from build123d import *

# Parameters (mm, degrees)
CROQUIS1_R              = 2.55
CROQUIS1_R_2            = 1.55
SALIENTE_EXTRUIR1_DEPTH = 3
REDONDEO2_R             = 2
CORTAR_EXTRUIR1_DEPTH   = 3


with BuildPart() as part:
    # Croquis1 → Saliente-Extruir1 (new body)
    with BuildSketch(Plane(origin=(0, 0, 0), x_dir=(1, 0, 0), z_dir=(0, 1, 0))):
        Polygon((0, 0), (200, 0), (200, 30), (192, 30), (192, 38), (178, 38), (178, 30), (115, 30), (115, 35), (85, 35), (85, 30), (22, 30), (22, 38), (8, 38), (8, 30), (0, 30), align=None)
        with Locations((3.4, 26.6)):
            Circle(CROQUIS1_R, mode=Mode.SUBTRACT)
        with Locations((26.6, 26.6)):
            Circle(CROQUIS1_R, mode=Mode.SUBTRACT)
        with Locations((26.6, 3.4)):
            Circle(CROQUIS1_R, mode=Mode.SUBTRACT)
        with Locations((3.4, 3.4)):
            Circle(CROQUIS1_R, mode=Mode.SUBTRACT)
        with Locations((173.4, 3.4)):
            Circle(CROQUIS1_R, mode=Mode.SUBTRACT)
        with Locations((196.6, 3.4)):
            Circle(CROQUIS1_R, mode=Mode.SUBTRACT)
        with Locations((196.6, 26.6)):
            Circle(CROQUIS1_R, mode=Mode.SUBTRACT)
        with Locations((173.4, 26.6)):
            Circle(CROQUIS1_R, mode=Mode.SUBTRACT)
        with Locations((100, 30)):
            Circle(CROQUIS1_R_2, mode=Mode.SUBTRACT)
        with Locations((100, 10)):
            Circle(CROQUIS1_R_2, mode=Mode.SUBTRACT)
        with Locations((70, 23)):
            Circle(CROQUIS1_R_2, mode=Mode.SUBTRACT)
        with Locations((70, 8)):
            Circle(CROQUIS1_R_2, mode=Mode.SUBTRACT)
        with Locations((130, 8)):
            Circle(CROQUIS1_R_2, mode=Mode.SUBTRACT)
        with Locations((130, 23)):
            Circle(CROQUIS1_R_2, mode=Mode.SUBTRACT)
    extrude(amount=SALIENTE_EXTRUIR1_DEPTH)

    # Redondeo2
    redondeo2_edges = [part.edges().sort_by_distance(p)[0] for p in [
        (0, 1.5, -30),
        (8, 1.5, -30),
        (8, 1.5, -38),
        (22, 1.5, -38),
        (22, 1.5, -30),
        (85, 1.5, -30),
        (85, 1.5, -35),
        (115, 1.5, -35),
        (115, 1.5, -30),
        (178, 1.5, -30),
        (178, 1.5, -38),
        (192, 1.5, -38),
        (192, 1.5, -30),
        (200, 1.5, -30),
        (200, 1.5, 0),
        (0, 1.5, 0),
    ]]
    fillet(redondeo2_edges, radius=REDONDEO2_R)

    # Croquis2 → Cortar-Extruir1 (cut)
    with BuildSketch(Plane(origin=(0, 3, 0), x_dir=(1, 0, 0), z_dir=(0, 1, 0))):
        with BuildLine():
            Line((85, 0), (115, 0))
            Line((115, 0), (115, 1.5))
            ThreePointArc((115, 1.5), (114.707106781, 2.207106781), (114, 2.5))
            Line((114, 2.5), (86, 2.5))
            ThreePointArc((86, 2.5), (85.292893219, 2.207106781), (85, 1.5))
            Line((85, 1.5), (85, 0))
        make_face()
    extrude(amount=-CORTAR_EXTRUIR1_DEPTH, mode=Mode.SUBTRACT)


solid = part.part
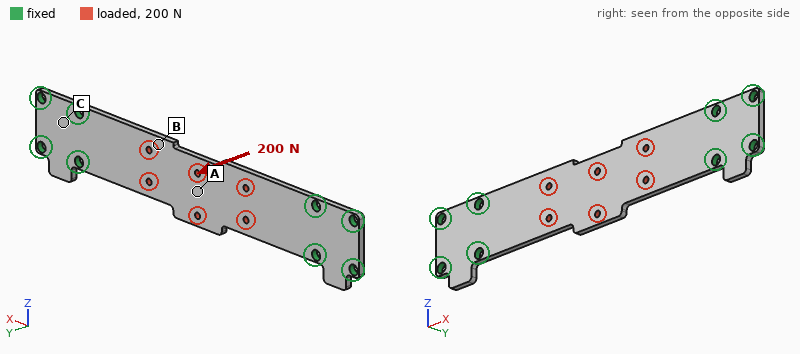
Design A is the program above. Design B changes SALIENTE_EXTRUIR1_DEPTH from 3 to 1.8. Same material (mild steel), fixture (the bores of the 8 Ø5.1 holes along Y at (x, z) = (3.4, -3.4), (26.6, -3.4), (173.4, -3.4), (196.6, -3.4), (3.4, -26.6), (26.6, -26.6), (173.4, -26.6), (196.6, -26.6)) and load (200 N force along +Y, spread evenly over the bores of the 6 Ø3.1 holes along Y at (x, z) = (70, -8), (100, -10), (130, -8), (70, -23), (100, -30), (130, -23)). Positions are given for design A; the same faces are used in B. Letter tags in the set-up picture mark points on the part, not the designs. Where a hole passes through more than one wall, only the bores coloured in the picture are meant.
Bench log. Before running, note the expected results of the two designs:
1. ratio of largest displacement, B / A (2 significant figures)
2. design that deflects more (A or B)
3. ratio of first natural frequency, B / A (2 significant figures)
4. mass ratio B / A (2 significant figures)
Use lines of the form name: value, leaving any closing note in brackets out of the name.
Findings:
ratio of largest displacement, B / A: 4.5
design that deflects more: B
ratio of first natural frequency, B / A: 0.61
mass ratio B / A: 0.60
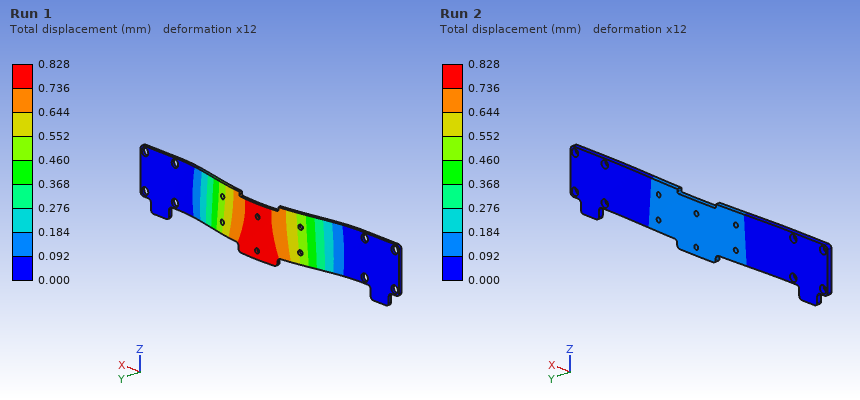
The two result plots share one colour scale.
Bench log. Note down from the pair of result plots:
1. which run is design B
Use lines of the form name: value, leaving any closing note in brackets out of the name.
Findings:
which run is design B: Run 1
